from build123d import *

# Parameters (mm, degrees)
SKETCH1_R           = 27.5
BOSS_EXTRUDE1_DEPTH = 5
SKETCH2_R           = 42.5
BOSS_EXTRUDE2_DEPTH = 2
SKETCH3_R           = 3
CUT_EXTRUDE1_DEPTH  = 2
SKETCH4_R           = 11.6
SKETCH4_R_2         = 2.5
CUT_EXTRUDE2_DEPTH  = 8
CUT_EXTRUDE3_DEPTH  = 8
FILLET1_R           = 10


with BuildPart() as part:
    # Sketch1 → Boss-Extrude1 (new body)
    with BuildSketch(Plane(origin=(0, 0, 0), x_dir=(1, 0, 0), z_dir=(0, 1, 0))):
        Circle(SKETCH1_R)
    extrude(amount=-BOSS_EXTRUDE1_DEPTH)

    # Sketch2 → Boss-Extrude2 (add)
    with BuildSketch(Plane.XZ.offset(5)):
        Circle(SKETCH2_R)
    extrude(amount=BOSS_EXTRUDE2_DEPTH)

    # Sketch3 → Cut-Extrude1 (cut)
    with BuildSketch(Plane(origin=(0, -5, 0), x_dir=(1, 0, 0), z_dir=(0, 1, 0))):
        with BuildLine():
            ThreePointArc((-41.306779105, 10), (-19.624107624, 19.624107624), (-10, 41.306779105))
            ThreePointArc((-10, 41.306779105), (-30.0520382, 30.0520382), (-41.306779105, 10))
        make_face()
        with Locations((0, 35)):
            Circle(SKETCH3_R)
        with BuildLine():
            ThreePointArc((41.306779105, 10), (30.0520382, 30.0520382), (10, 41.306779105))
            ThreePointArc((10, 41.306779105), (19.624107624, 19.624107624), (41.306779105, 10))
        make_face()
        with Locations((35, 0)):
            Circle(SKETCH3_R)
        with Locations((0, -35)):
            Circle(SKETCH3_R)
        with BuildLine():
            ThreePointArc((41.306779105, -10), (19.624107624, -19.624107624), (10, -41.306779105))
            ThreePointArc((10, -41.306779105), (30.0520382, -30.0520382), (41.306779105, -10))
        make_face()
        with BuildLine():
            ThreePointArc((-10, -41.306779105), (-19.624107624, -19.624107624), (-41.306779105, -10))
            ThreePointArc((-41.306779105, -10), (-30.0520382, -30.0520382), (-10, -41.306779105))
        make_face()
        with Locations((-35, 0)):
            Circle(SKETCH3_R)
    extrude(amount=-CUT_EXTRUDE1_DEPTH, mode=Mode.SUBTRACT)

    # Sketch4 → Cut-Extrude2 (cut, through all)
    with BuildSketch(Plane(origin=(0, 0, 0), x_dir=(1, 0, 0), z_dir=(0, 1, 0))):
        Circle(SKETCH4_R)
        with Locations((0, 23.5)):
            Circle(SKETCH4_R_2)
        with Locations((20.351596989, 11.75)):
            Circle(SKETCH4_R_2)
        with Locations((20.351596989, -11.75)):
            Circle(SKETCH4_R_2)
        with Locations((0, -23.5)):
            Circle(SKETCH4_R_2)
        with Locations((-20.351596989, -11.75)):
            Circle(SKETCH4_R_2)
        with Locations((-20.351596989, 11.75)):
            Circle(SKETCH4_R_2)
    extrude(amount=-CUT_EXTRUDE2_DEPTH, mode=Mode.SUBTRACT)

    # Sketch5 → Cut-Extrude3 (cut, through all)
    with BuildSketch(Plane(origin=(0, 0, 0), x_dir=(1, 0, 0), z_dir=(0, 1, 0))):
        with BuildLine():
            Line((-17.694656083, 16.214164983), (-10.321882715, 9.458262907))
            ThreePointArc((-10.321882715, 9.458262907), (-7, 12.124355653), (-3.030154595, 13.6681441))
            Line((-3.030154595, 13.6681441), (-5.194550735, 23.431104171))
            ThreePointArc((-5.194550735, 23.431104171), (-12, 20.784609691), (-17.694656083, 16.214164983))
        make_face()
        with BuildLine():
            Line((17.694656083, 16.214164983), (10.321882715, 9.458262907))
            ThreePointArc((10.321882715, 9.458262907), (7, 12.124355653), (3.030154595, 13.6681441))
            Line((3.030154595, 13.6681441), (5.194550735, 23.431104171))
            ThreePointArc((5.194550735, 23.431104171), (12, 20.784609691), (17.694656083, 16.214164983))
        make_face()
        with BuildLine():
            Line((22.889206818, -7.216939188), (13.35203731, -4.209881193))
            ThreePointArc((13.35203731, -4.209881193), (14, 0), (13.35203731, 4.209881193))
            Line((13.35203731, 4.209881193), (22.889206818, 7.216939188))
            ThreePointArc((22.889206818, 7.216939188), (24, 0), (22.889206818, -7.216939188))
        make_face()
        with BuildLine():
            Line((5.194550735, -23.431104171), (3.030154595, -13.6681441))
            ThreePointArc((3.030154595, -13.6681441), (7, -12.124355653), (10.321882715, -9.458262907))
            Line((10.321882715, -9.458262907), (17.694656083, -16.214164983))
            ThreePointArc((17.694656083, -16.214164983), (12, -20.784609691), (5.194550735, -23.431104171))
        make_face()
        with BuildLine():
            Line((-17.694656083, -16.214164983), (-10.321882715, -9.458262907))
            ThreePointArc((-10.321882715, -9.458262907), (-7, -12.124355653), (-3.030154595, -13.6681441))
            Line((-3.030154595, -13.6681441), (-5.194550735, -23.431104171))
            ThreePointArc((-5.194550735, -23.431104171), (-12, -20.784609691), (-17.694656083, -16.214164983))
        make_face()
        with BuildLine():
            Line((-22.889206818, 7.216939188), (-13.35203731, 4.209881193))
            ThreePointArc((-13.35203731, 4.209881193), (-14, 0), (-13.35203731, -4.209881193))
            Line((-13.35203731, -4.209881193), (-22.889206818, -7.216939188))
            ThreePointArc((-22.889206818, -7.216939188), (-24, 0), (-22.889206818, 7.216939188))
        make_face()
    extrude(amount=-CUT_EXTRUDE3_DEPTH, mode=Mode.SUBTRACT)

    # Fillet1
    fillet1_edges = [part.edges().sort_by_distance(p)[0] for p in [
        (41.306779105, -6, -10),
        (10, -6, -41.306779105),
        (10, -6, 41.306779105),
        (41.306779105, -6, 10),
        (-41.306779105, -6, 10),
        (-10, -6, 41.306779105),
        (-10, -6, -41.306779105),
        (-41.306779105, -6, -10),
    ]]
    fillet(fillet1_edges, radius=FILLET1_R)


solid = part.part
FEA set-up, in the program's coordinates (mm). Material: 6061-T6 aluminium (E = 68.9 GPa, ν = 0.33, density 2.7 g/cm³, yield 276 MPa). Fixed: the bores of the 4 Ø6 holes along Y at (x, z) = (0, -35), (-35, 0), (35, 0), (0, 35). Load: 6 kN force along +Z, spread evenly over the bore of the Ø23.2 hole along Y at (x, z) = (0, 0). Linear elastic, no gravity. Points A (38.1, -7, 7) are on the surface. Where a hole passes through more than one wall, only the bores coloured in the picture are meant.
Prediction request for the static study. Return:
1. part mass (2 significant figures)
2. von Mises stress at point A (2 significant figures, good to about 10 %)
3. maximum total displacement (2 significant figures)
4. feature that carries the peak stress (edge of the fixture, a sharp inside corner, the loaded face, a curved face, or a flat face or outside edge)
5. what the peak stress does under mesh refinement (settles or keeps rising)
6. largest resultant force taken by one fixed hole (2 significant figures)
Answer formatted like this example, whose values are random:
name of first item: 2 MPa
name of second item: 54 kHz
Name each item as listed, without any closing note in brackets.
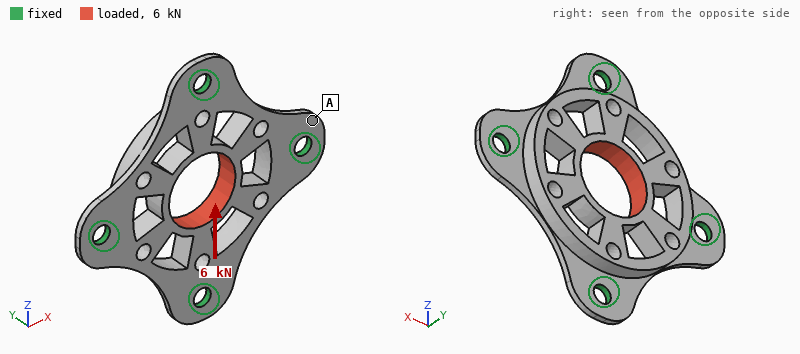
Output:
part mass: 29 g
von Mises stress at point A: 25 MPa
maximum total displacement: 55 µm
feature that carries the peak stress: edge of the fixture
what the peak stress does under mesh refinement: keeps rising
largest resultant force taken by one fixed hole: 2.0 kN
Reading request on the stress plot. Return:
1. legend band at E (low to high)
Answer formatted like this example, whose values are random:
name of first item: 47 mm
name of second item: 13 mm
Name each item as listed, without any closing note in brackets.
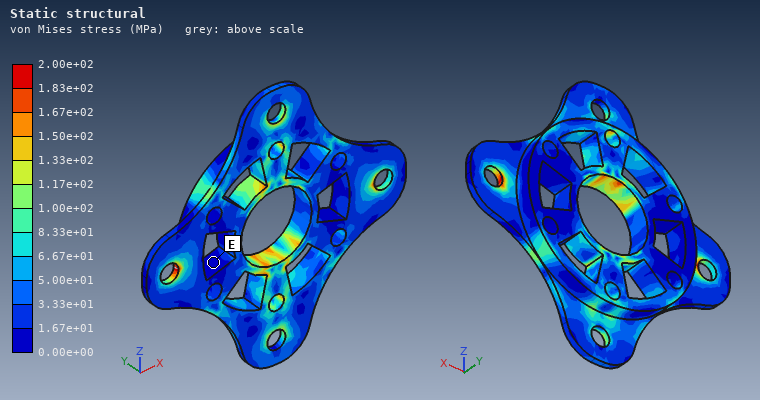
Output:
legend band at E: 0.00e+00 to 1.67e+01 MPa
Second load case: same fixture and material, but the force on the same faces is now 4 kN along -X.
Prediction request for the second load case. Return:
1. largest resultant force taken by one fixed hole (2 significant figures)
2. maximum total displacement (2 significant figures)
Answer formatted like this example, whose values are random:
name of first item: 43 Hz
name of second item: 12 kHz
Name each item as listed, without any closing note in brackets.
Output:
largest resultant force taken by one fixed hole: 1.4 kN
maximum total displacement: 28 µm
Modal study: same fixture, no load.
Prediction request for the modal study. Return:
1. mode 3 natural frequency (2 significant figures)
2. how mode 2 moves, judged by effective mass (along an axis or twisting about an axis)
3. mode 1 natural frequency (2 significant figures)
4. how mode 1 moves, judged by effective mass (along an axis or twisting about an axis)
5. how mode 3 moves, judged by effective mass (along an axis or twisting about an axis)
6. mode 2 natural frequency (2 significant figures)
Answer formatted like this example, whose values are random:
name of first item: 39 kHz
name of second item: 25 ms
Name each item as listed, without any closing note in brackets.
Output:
mode 3 natural frequency: 8900 Hz
how mode 2 moves, judged by effective mass: twisting about X
mode 1 natural frequency: 6200 Hz
how mode 1 moves, judged by effective mass: along Y
how mode 3 moves, judged by effective mass: twisting about Z
mode 2 natural frequency: 8500 Hz
